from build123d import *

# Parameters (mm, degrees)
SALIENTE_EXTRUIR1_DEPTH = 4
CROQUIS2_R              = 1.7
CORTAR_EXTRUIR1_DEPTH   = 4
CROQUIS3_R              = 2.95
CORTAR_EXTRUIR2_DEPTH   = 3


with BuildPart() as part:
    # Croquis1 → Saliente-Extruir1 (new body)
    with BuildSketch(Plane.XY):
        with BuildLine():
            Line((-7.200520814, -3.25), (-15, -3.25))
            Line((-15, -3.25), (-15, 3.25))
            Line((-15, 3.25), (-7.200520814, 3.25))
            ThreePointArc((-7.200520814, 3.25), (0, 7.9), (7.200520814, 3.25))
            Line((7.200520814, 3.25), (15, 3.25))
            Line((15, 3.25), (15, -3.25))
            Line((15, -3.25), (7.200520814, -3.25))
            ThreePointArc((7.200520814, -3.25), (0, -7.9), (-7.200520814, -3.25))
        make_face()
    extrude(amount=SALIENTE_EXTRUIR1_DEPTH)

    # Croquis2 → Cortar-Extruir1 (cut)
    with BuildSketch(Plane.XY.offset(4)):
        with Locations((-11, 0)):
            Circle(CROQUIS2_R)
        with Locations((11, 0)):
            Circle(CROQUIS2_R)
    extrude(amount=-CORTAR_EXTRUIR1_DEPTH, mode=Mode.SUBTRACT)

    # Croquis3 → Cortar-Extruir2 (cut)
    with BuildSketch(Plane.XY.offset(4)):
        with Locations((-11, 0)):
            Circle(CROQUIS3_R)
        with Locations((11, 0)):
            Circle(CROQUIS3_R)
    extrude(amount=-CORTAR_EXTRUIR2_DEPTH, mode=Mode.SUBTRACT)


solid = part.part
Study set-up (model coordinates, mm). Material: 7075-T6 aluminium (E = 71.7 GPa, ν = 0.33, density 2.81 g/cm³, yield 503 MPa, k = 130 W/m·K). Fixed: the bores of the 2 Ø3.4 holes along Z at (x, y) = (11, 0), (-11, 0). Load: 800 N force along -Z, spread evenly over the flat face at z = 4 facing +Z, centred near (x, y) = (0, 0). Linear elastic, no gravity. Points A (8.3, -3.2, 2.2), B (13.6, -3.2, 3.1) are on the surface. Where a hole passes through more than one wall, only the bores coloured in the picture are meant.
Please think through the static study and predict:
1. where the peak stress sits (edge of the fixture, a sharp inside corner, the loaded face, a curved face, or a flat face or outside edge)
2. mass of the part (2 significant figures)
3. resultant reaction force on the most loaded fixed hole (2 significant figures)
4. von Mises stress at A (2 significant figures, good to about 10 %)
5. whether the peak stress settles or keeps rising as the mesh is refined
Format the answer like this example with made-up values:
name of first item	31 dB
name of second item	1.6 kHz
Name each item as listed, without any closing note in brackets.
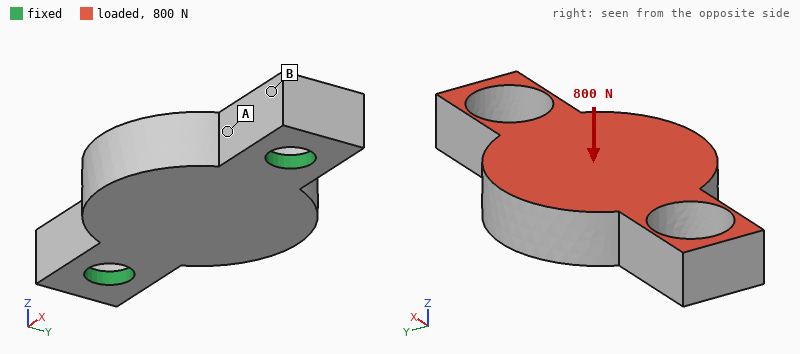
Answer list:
where the peak stress sits	edge of the fixture
mass of the part	2.8 g
resultant reaction force on the most loaded fixed hole	530 N
von Mises stress at A	49 MPa
whether the peak stress settles or keeps rising as the mesh is refined	keeps rising
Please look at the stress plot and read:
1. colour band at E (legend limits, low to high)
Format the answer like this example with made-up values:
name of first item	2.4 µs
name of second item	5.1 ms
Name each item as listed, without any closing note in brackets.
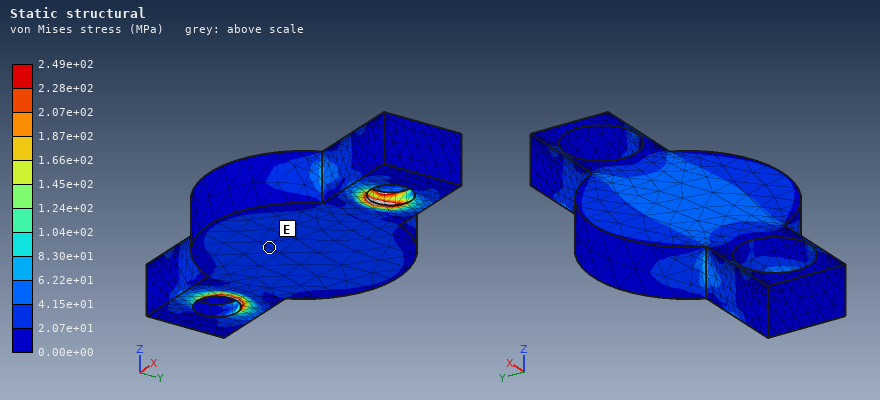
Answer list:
colour band at E	2.07e+01 to 4.15e+01 MPa
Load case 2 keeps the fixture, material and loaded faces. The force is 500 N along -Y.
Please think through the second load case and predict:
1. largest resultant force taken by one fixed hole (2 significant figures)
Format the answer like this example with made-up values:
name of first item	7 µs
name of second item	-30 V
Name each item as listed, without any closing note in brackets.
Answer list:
largest resultant force taken by one fixed hole	250 N
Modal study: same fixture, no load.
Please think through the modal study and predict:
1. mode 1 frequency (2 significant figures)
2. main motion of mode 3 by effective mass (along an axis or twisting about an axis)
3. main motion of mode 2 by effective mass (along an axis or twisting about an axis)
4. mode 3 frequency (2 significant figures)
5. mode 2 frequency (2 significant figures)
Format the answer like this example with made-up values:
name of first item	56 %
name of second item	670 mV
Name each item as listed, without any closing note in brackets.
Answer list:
mode 1 frequency	13 kHz
main motion of mode 3 by effective mass	along Y
main motion of mode 2 by effective mass	along Z
mode 3 frequency	35 kHz
mode 2 frequency	21 kHz
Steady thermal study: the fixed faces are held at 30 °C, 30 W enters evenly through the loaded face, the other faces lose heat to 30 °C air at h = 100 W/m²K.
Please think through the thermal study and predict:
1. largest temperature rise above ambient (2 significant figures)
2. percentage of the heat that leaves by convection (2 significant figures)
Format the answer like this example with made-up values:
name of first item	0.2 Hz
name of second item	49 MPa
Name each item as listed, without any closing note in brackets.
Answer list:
largest temperature rise above ambient	41 K
percentage of the heat that leaves by convection	5.7 %
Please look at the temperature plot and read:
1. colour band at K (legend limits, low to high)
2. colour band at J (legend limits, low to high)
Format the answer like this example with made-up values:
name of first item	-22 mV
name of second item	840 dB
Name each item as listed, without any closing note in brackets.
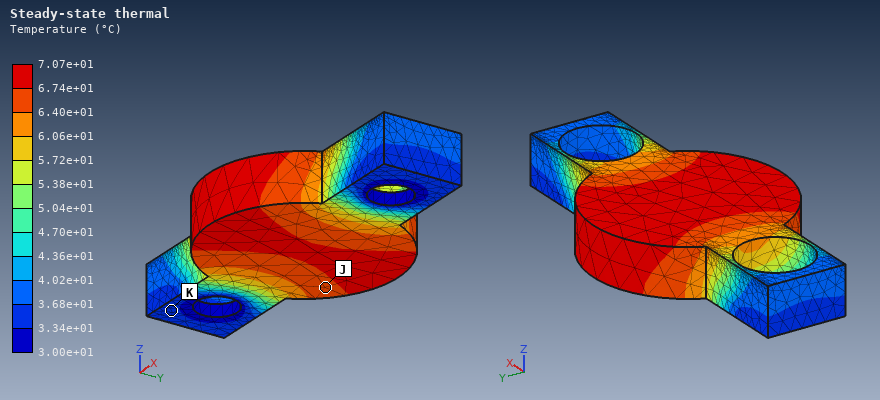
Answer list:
colour band at K	3.34e+01 to 3.68e+01 °C
colour band at J	6.40e+01 to 6.74e+01 °C
